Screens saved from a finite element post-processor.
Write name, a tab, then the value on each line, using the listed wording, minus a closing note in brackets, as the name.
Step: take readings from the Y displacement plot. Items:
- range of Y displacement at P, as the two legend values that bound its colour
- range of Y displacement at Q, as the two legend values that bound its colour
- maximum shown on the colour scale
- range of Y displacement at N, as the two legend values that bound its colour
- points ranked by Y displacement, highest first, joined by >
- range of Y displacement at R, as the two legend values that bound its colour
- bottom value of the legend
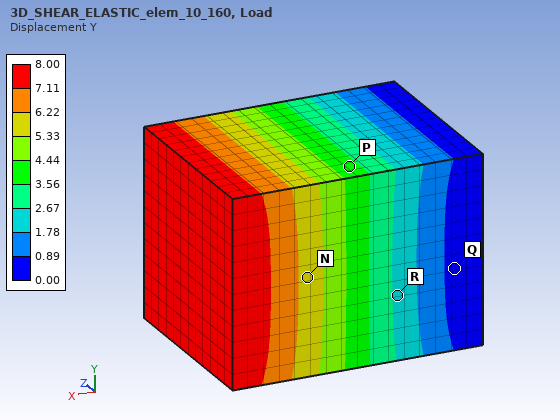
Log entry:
range of Y displacement at P, as the two legend values that bound its colour	3.56 to 4.44
range of Y displacement at Q, as the two legend values that bound its colour	0.00 to 0.89
maximum shown on the colour scale	8.00
range of Y displacement at N, as the two legend values that bound its colour	5.33 to 6.22
points ranked by Y displacement, highest first, joined by >	N > P > R > Q
range of Y displacement at R, as the two legend values that bound its colour	1.78 to 2.67
bottom value of the legend	0.00
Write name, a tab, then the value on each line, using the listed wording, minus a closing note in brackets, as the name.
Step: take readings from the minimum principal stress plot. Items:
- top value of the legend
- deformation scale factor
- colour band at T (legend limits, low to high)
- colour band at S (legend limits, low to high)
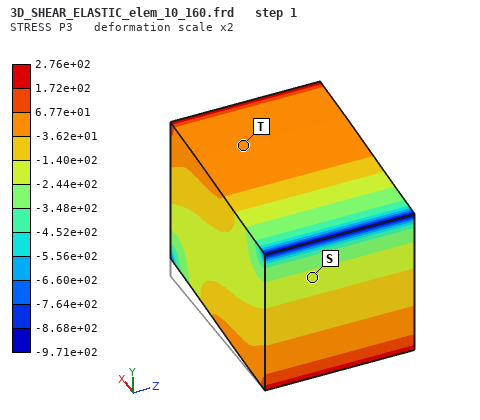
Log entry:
top value of the legend	2.76e+02
deformation scale factor	2
colour band at T	-3.62e+01 to 6.77e+01
colour band at S	-2.44e+02 to -1.40e+02
